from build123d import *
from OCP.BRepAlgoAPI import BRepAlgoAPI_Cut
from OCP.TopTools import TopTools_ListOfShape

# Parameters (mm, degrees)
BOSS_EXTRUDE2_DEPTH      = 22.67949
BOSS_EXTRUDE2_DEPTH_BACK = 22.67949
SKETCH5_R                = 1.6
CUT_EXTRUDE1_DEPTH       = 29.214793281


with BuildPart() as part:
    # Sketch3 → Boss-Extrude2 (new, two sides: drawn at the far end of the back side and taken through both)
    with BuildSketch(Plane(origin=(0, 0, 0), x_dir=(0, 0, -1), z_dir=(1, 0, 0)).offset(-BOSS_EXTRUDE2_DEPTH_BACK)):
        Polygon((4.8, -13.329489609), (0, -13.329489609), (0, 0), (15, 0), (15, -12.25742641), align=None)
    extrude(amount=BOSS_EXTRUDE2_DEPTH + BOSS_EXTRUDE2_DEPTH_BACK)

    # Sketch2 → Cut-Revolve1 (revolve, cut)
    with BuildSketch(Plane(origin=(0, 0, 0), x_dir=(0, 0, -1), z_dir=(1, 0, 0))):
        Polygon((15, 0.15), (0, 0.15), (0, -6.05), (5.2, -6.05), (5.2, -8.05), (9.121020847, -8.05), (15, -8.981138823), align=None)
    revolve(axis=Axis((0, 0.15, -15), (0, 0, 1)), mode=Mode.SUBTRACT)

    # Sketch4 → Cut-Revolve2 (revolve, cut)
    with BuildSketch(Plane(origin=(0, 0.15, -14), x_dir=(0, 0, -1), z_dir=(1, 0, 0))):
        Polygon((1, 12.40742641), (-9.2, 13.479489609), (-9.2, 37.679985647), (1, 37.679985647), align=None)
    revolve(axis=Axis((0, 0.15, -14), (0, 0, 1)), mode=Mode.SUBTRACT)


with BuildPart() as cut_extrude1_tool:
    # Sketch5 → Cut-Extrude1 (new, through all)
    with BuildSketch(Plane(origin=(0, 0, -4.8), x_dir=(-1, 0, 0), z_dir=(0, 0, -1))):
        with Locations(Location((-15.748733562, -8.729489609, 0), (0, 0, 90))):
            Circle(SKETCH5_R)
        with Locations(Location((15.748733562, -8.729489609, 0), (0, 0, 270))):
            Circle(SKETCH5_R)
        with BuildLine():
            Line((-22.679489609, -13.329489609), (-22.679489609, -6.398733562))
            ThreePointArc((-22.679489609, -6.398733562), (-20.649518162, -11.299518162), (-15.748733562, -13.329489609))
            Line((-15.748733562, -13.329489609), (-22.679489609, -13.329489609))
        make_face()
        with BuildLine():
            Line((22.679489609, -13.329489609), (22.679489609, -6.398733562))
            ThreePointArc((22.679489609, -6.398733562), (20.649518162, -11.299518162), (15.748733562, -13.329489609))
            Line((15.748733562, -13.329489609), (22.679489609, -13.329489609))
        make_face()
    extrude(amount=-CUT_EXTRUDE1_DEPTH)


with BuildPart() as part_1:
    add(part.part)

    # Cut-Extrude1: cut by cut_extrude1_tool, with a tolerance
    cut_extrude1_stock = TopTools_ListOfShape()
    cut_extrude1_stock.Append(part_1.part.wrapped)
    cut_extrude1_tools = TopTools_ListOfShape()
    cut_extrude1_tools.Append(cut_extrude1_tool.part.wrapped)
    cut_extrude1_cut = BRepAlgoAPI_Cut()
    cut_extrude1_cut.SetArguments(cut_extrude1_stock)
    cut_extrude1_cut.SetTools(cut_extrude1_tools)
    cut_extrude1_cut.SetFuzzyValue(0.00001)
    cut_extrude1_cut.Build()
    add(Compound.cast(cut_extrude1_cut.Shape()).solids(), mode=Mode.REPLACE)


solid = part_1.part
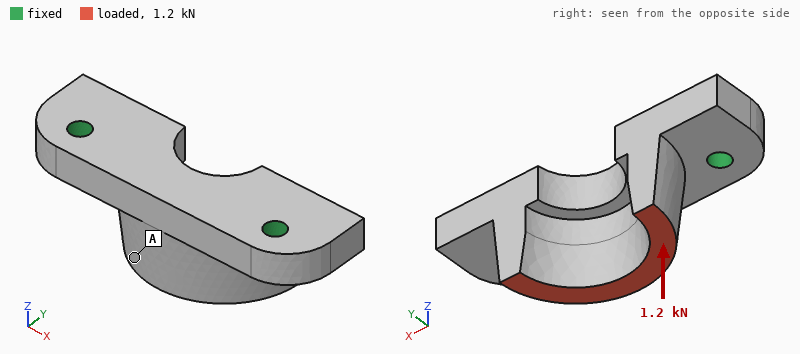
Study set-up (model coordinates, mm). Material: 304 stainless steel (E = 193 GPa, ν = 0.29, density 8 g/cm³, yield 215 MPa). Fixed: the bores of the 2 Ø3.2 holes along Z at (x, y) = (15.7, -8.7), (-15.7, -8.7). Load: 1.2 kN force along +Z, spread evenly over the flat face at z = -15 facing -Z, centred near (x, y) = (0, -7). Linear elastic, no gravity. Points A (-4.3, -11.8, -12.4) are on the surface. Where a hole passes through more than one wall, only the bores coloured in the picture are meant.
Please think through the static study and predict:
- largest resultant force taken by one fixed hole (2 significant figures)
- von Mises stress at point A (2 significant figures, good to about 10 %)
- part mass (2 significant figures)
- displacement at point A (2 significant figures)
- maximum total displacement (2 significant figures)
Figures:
630 N
13 MPa
32 g
3.1 µm
4.0 µm
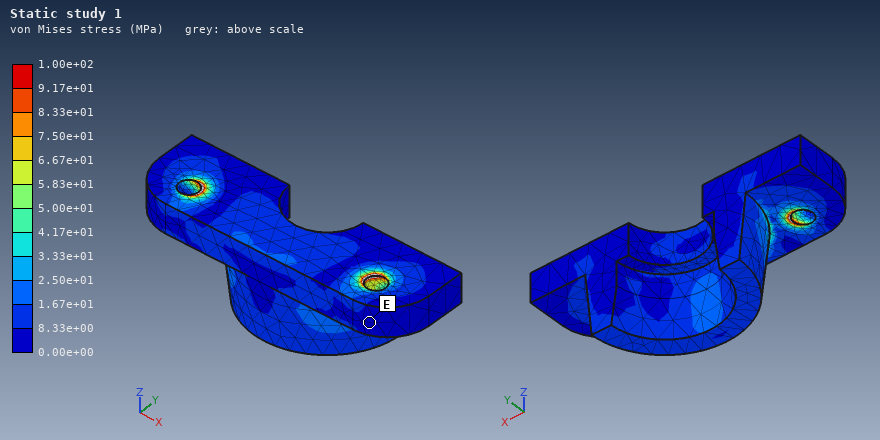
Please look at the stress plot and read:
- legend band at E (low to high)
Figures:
0.00e+00 to 8.33e+00 MPa
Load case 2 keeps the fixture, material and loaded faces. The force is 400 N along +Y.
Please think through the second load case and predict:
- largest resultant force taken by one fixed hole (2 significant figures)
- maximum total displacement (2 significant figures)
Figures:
200 N
9.9 µm
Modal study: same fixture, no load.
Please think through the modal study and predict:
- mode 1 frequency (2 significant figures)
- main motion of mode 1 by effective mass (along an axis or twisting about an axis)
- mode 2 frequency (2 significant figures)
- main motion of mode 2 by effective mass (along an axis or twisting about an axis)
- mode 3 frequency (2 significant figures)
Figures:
13 kHz
along Y
21 kHz
along Z
24 kHz
